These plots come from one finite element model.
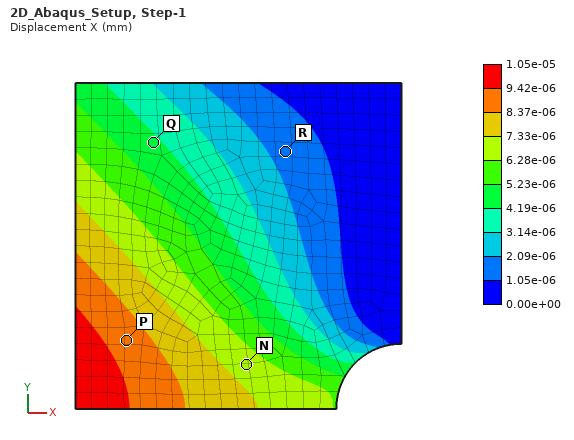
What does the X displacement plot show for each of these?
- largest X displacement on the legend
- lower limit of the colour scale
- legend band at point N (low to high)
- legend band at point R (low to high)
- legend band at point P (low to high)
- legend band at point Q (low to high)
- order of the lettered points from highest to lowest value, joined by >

1.05e-05 mm
0.00e+00 mm
6.28e-06 to 7.33e-06 mm
1.05e-06 to 2.09e-06 mm
8.37e-06 to 9.42e-06 mm
4.19e-06 to 5.23e-06 mm
P > N > Q > R
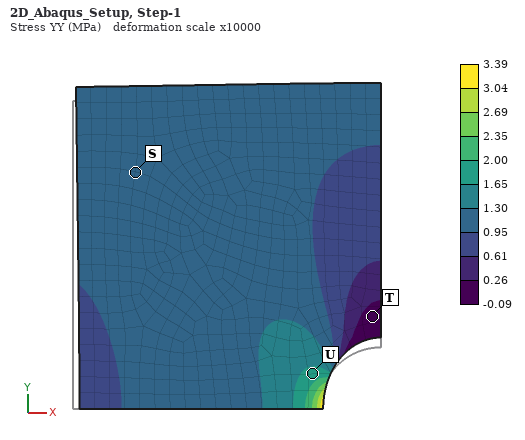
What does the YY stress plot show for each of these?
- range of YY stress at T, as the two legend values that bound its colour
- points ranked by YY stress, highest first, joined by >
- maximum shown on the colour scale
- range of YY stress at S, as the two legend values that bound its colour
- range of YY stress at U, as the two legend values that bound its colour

-0.09 to 0.26 MPa
U > S > T
3.39 MPa
0.95 to 1.30 MPa
1.65 to 2.00 MPa
